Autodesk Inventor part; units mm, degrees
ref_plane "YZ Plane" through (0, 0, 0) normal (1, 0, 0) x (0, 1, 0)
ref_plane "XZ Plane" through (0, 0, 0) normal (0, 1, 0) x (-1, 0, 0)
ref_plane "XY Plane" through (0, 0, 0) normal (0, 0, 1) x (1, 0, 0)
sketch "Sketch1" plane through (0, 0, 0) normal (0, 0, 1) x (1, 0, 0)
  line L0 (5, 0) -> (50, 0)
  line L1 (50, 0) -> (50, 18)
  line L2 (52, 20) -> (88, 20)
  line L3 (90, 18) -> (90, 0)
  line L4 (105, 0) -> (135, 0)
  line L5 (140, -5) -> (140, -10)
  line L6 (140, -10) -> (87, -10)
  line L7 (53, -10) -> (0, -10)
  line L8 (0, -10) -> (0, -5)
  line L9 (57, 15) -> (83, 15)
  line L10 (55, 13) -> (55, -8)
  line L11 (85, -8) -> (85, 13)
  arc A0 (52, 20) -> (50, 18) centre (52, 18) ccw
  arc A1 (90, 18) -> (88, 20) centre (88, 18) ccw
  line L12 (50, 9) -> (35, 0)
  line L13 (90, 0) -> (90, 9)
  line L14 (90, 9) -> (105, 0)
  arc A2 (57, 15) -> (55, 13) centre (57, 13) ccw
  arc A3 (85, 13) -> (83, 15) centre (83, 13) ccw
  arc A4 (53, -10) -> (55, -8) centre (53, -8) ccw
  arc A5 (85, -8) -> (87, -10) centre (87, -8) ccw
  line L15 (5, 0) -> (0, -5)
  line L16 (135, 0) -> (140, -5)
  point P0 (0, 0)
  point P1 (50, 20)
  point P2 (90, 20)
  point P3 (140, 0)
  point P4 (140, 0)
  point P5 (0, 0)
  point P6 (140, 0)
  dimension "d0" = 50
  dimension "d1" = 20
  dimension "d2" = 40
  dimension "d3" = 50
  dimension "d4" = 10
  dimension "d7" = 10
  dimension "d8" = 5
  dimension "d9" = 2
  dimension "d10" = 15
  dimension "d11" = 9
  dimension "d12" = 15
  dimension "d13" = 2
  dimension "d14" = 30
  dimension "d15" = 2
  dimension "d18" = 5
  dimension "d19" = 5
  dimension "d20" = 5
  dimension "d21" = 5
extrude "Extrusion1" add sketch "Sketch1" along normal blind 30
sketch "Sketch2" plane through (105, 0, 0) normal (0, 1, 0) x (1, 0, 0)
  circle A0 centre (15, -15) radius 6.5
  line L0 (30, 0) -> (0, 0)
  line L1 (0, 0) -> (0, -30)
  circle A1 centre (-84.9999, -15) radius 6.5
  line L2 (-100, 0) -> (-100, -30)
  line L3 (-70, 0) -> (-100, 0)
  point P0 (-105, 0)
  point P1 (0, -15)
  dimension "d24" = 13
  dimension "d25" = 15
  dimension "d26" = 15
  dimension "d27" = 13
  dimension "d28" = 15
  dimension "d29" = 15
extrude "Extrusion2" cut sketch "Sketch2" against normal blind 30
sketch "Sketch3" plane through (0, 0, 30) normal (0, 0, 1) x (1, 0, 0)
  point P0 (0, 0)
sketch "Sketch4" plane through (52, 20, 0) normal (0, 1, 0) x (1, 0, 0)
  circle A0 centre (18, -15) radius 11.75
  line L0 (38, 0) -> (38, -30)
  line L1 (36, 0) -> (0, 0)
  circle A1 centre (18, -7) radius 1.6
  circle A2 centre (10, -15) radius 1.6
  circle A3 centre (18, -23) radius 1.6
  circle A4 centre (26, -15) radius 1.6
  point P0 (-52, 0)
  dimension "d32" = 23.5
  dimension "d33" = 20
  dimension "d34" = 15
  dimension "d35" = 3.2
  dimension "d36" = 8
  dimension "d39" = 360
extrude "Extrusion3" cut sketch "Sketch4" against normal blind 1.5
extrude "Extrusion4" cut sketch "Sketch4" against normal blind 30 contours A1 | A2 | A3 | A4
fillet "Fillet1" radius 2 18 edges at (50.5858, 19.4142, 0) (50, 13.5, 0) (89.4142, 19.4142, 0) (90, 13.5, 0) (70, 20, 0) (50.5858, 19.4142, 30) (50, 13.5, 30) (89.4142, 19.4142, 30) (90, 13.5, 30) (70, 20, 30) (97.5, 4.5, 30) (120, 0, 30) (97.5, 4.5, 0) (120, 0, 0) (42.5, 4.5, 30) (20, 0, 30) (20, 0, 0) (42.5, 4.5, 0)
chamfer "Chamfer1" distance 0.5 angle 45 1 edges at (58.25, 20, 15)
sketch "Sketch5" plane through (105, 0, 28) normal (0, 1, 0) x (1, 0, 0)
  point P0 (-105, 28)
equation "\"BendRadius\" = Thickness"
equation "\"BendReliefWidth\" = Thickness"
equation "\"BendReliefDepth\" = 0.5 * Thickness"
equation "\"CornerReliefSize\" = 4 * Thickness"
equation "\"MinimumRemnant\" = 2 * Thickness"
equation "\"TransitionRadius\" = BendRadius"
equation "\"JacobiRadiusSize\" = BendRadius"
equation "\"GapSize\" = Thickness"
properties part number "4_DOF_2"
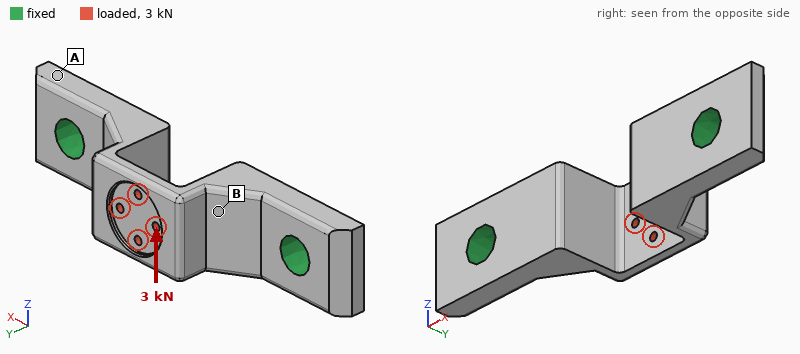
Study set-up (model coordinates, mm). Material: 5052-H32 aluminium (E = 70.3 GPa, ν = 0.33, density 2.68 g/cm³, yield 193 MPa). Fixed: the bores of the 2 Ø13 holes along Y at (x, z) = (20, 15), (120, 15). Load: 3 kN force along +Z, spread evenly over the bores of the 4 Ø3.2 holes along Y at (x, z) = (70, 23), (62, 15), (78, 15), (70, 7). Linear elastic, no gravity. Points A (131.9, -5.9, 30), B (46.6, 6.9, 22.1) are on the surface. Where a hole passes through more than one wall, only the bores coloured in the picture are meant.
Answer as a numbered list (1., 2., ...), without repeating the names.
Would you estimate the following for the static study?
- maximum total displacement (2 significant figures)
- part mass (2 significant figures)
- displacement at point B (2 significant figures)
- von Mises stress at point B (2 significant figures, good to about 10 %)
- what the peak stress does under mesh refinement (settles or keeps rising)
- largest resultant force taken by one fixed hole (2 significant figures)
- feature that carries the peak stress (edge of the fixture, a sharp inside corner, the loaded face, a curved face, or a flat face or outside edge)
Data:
1. 92 µm
2. 120 g
3. 43 µm
4. 30 MPa
5. keeps rising
6. 1.5 kN
7. edge of the fixture
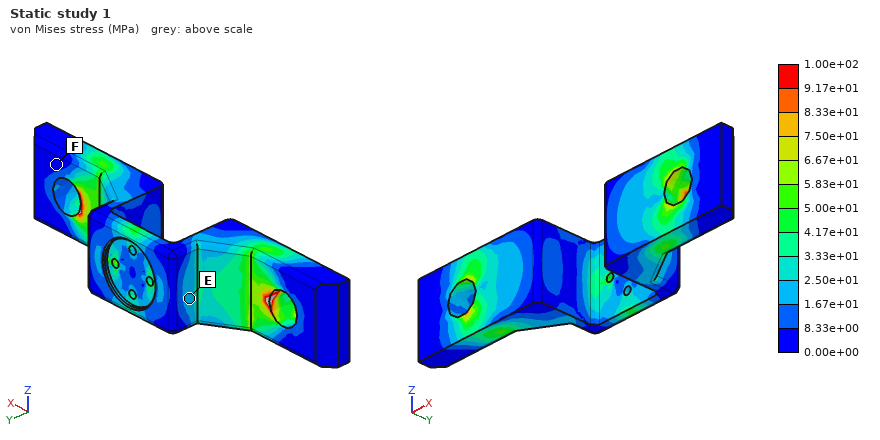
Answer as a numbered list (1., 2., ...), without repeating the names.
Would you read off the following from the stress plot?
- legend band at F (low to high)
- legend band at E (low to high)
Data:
1. 0.00e+00 to 8.33e+00 MPa
2. 1.67e+01 to 2.50e+01 MPa
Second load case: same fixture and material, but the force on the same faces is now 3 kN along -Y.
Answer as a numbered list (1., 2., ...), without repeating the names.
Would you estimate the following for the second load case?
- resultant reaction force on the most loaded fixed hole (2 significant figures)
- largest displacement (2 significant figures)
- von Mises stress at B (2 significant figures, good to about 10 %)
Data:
1. 2.3 kN
2. 67 µm
3. 21 MPa
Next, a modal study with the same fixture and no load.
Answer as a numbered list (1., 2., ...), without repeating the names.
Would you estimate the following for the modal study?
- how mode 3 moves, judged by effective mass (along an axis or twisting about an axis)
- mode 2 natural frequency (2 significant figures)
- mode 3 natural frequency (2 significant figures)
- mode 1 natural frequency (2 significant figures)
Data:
1. along Y
2. 6100 Hz
3. 7600 Hz
4. 6000 Hz
